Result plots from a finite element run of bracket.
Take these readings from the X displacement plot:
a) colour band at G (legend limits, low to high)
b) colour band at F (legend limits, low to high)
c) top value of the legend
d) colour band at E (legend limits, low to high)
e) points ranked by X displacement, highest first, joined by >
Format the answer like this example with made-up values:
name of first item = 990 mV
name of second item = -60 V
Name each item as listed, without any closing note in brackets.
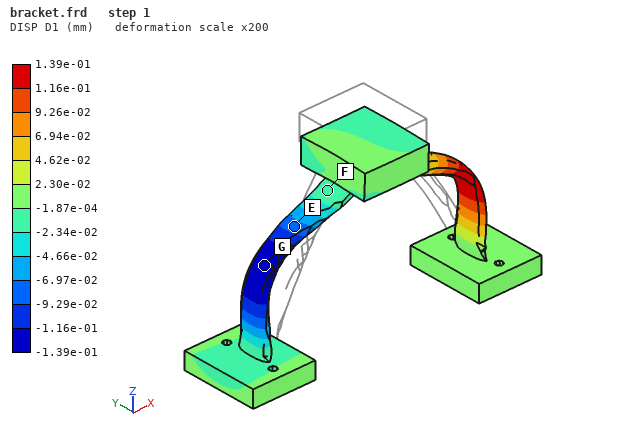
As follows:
colour band at G = -1.39e-01 to -1.16e-01 mm
colour band at F = -2.34e-02 to -1.87e-04 mm
top value of the legend = 1.39e-01 mm
colour band at E = -9.29e-02 to -6.97e-02 mm
points ranked by X displacement, highest first, joined by > = F > E > G
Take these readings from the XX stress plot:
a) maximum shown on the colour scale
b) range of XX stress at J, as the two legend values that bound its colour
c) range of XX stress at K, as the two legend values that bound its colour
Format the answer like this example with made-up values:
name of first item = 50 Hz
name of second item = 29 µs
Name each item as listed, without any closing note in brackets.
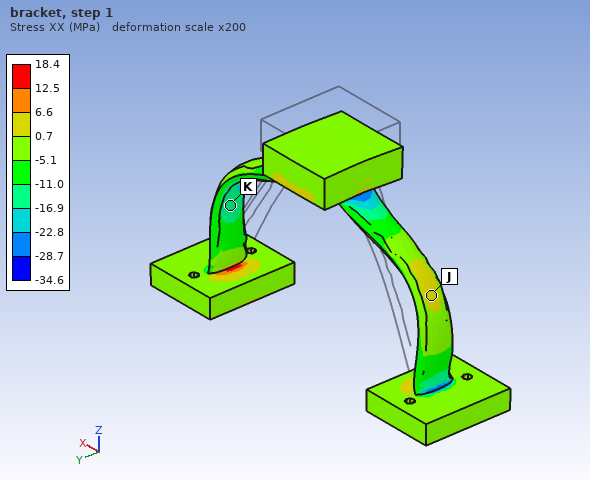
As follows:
maximum shown on the colour scale = 18.4 MPa
range of XX stress at J, as the two legend values that bound its colour = 0.7 to 6.6 MPa
range of XX stress at K, as the two legend values that bound its colour = -16.9 to -11.0 MPa
